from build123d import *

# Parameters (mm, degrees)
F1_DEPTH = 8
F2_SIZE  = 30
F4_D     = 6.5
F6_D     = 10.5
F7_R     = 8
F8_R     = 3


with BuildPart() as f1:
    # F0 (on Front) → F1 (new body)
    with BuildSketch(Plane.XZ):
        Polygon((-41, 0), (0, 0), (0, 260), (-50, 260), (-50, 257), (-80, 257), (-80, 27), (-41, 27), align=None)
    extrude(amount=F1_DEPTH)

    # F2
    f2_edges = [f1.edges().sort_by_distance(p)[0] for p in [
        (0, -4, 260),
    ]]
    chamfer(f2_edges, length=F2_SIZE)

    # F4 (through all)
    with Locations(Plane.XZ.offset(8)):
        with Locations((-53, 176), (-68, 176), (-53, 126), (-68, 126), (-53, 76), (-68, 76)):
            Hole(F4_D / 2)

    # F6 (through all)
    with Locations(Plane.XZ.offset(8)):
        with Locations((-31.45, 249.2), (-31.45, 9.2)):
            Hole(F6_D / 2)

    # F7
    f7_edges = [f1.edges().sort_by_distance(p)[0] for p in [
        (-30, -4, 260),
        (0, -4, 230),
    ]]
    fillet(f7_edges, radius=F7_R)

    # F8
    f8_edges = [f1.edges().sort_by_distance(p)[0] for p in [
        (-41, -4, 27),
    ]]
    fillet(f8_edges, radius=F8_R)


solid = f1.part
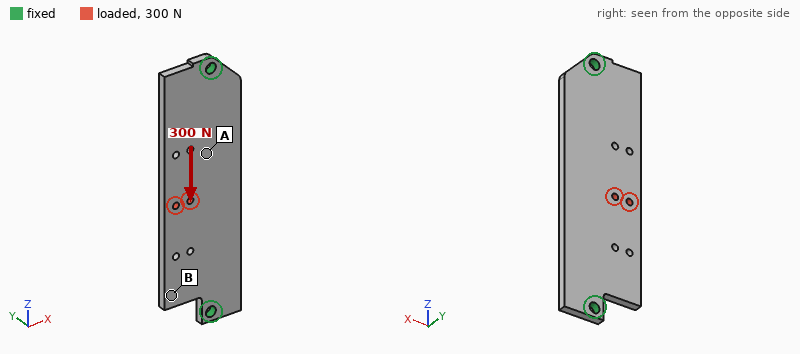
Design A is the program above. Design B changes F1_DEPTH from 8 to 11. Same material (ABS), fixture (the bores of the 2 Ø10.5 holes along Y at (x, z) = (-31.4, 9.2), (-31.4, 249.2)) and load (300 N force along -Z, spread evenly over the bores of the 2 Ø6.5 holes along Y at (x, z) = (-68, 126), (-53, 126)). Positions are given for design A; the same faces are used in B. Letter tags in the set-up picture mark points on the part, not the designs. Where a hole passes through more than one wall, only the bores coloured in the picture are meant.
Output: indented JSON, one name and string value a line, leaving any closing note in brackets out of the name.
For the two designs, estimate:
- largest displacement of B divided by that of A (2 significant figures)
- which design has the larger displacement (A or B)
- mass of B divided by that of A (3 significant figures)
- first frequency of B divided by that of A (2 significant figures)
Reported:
{
  "largest displacement of B divided by that of A": "0.73",
  "which design has the larger displacement": "A",
  "mass of B divided by that of A": "1.37",
  "first frequency of B divided by that of A": "1.3"
}
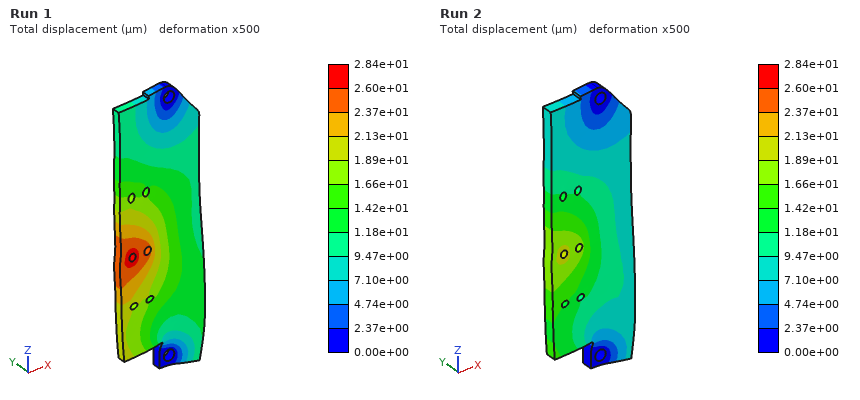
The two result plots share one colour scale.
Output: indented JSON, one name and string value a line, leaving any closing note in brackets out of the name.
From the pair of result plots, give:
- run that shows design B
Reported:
{
  "run that shows design B": "Run 2"
}
